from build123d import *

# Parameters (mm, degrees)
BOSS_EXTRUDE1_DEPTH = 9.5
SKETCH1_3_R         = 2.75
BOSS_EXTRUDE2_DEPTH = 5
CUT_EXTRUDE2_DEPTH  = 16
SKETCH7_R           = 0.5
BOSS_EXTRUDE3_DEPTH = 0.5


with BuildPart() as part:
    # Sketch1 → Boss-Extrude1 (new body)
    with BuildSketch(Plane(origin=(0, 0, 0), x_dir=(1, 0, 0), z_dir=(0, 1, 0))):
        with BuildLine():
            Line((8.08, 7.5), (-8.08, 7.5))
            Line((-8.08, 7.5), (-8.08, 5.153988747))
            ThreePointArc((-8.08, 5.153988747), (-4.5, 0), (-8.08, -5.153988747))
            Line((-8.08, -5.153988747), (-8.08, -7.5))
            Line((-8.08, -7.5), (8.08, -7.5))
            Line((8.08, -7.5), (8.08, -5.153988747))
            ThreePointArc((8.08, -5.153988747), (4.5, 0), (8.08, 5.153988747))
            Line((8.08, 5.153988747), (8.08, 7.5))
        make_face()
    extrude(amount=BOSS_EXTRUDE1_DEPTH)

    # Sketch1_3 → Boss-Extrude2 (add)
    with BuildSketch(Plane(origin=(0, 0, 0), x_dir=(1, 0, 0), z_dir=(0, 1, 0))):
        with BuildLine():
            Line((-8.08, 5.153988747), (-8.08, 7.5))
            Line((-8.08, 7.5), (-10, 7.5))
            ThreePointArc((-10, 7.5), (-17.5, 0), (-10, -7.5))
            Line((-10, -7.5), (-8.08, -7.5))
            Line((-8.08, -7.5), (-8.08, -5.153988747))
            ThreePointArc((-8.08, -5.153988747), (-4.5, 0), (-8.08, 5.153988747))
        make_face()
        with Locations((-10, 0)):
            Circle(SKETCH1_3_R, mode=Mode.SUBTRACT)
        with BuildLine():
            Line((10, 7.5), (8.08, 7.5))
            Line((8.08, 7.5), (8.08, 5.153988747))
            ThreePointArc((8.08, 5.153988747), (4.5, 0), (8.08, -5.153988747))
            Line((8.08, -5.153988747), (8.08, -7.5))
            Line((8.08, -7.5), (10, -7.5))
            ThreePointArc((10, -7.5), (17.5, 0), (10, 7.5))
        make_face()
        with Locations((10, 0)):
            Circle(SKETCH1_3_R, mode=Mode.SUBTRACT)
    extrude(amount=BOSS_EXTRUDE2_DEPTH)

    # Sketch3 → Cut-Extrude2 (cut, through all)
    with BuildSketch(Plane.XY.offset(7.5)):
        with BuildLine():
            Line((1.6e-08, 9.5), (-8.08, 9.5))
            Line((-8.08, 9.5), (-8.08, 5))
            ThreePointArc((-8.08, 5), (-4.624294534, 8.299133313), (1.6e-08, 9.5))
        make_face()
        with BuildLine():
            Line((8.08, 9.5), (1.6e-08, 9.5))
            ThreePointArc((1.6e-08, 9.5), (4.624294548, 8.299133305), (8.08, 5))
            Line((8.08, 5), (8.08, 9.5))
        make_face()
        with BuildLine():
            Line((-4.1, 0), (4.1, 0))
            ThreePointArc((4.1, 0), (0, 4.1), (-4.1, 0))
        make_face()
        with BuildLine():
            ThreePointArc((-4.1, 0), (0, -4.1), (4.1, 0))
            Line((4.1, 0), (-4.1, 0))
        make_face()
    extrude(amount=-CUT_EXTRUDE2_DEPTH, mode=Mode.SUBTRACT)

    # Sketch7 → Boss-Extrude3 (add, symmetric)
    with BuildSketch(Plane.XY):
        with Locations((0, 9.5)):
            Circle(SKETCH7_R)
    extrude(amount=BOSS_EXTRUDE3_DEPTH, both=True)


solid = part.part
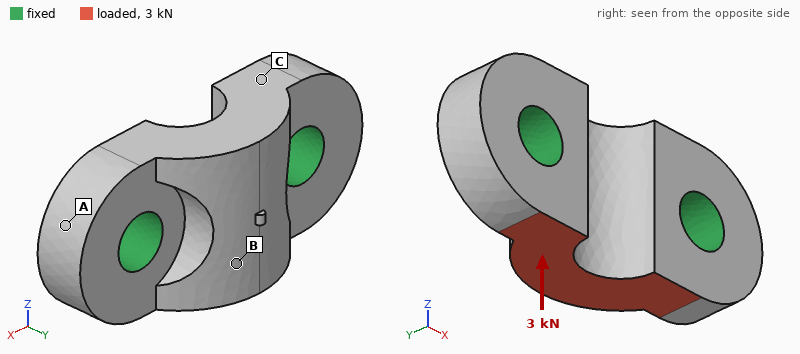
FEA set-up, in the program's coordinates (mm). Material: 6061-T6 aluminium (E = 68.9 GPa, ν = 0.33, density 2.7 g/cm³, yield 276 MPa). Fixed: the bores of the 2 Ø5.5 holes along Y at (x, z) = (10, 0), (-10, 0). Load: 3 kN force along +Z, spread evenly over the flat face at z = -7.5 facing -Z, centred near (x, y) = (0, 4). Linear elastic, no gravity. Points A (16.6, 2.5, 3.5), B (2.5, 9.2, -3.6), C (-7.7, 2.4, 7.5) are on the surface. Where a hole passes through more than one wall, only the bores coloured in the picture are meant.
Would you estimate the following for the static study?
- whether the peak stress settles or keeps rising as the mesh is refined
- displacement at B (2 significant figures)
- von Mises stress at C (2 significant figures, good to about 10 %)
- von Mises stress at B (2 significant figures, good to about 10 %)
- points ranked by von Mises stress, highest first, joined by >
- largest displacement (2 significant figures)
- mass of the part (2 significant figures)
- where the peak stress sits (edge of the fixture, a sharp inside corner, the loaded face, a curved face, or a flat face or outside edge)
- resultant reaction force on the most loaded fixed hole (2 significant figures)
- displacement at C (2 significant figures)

keeps rising
12 µm
23 MPa
33 MPa
B > C > A
17 µm
6.6 g
edge of the fixture
1.5 kN
4.1 µm
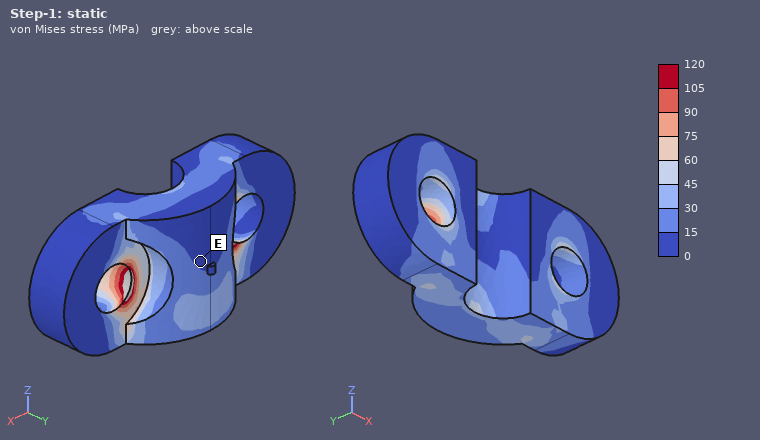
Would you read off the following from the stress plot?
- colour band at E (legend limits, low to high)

0 to 15 MPa
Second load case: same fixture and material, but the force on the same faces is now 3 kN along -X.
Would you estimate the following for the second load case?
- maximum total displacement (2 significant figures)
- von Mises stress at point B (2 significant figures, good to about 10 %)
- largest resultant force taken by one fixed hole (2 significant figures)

11 µm
16 MPa
1.7 kN
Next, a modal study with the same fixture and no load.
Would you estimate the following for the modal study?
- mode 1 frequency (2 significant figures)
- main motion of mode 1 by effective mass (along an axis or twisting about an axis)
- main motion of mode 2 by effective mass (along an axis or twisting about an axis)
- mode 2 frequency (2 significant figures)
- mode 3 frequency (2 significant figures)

38 kHz
along Z
along Y
57 kHz
75 kHz
